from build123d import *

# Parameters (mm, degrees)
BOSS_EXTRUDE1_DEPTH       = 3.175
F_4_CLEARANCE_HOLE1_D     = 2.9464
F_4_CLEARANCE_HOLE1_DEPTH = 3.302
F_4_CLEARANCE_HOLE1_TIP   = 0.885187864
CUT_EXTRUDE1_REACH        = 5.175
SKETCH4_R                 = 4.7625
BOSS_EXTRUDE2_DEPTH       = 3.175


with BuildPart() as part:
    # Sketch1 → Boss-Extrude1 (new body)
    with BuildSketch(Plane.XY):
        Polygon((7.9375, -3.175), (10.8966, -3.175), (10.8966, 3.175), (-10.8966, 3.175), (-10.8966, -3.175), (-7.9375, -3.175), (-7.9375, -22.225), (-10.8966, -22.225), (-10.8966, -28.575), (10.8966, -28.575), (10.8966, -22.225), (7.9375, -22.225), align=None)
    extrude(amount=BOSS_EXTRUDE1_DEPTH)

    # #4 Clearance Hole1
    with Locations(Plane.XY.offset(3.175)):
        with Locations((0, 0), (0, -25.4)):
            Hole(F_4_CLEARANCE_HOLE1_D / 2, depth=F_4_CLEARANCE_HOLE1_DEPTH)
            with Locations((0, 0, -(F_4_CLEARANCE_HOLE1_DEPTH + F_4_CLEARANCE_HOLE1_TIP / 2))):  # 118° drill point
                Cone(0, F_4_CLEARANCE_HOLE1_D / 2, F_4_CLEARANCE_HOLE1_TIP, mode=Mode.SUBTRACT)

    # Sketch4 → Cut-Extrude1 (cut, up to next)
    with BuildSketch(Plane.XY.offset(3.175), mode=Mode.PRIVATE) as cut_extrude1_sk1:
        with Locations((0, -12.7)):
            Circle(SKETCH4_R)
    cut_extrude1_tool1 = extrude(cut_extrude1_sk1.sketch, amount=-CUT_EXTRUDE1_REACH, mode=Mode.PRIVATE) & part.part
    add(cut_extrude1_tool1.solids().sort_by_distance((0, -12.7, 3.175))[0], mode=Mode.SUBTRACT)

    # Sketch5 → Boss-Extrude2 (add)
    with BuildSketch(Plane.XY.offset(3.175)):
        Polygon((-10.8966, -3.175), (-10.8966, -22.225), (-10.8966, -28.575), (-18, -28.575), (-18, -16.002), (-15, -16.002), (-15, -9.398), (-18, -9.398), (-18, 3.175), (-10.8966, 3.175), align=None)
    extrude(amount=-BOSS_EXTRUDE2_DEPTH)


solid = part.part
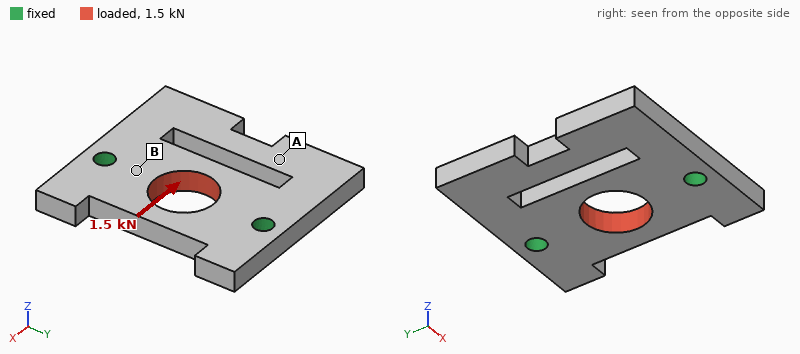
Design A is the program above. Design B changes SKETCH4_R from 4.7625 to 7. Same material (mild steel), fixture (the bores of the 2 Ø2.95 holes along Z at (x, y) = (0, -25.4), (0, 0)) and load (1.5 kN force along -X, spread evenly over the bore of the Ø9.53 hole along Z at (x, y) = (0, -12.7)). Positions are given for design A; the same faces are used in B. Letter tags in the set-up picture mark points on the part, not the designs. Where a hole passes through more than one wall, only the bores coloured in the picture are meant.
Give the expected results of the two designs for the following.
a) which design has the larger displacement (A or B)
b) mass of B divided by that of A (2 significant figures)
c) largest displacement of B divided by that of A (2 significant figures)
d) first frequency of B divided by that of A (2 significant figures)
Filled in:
B
0.88
2.1
0.98
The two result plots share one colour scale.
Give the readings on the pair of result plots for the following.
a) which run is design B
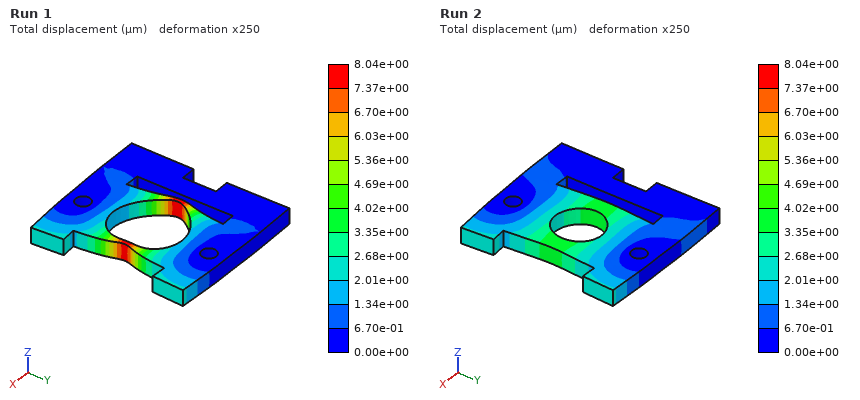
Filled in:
Run 1
